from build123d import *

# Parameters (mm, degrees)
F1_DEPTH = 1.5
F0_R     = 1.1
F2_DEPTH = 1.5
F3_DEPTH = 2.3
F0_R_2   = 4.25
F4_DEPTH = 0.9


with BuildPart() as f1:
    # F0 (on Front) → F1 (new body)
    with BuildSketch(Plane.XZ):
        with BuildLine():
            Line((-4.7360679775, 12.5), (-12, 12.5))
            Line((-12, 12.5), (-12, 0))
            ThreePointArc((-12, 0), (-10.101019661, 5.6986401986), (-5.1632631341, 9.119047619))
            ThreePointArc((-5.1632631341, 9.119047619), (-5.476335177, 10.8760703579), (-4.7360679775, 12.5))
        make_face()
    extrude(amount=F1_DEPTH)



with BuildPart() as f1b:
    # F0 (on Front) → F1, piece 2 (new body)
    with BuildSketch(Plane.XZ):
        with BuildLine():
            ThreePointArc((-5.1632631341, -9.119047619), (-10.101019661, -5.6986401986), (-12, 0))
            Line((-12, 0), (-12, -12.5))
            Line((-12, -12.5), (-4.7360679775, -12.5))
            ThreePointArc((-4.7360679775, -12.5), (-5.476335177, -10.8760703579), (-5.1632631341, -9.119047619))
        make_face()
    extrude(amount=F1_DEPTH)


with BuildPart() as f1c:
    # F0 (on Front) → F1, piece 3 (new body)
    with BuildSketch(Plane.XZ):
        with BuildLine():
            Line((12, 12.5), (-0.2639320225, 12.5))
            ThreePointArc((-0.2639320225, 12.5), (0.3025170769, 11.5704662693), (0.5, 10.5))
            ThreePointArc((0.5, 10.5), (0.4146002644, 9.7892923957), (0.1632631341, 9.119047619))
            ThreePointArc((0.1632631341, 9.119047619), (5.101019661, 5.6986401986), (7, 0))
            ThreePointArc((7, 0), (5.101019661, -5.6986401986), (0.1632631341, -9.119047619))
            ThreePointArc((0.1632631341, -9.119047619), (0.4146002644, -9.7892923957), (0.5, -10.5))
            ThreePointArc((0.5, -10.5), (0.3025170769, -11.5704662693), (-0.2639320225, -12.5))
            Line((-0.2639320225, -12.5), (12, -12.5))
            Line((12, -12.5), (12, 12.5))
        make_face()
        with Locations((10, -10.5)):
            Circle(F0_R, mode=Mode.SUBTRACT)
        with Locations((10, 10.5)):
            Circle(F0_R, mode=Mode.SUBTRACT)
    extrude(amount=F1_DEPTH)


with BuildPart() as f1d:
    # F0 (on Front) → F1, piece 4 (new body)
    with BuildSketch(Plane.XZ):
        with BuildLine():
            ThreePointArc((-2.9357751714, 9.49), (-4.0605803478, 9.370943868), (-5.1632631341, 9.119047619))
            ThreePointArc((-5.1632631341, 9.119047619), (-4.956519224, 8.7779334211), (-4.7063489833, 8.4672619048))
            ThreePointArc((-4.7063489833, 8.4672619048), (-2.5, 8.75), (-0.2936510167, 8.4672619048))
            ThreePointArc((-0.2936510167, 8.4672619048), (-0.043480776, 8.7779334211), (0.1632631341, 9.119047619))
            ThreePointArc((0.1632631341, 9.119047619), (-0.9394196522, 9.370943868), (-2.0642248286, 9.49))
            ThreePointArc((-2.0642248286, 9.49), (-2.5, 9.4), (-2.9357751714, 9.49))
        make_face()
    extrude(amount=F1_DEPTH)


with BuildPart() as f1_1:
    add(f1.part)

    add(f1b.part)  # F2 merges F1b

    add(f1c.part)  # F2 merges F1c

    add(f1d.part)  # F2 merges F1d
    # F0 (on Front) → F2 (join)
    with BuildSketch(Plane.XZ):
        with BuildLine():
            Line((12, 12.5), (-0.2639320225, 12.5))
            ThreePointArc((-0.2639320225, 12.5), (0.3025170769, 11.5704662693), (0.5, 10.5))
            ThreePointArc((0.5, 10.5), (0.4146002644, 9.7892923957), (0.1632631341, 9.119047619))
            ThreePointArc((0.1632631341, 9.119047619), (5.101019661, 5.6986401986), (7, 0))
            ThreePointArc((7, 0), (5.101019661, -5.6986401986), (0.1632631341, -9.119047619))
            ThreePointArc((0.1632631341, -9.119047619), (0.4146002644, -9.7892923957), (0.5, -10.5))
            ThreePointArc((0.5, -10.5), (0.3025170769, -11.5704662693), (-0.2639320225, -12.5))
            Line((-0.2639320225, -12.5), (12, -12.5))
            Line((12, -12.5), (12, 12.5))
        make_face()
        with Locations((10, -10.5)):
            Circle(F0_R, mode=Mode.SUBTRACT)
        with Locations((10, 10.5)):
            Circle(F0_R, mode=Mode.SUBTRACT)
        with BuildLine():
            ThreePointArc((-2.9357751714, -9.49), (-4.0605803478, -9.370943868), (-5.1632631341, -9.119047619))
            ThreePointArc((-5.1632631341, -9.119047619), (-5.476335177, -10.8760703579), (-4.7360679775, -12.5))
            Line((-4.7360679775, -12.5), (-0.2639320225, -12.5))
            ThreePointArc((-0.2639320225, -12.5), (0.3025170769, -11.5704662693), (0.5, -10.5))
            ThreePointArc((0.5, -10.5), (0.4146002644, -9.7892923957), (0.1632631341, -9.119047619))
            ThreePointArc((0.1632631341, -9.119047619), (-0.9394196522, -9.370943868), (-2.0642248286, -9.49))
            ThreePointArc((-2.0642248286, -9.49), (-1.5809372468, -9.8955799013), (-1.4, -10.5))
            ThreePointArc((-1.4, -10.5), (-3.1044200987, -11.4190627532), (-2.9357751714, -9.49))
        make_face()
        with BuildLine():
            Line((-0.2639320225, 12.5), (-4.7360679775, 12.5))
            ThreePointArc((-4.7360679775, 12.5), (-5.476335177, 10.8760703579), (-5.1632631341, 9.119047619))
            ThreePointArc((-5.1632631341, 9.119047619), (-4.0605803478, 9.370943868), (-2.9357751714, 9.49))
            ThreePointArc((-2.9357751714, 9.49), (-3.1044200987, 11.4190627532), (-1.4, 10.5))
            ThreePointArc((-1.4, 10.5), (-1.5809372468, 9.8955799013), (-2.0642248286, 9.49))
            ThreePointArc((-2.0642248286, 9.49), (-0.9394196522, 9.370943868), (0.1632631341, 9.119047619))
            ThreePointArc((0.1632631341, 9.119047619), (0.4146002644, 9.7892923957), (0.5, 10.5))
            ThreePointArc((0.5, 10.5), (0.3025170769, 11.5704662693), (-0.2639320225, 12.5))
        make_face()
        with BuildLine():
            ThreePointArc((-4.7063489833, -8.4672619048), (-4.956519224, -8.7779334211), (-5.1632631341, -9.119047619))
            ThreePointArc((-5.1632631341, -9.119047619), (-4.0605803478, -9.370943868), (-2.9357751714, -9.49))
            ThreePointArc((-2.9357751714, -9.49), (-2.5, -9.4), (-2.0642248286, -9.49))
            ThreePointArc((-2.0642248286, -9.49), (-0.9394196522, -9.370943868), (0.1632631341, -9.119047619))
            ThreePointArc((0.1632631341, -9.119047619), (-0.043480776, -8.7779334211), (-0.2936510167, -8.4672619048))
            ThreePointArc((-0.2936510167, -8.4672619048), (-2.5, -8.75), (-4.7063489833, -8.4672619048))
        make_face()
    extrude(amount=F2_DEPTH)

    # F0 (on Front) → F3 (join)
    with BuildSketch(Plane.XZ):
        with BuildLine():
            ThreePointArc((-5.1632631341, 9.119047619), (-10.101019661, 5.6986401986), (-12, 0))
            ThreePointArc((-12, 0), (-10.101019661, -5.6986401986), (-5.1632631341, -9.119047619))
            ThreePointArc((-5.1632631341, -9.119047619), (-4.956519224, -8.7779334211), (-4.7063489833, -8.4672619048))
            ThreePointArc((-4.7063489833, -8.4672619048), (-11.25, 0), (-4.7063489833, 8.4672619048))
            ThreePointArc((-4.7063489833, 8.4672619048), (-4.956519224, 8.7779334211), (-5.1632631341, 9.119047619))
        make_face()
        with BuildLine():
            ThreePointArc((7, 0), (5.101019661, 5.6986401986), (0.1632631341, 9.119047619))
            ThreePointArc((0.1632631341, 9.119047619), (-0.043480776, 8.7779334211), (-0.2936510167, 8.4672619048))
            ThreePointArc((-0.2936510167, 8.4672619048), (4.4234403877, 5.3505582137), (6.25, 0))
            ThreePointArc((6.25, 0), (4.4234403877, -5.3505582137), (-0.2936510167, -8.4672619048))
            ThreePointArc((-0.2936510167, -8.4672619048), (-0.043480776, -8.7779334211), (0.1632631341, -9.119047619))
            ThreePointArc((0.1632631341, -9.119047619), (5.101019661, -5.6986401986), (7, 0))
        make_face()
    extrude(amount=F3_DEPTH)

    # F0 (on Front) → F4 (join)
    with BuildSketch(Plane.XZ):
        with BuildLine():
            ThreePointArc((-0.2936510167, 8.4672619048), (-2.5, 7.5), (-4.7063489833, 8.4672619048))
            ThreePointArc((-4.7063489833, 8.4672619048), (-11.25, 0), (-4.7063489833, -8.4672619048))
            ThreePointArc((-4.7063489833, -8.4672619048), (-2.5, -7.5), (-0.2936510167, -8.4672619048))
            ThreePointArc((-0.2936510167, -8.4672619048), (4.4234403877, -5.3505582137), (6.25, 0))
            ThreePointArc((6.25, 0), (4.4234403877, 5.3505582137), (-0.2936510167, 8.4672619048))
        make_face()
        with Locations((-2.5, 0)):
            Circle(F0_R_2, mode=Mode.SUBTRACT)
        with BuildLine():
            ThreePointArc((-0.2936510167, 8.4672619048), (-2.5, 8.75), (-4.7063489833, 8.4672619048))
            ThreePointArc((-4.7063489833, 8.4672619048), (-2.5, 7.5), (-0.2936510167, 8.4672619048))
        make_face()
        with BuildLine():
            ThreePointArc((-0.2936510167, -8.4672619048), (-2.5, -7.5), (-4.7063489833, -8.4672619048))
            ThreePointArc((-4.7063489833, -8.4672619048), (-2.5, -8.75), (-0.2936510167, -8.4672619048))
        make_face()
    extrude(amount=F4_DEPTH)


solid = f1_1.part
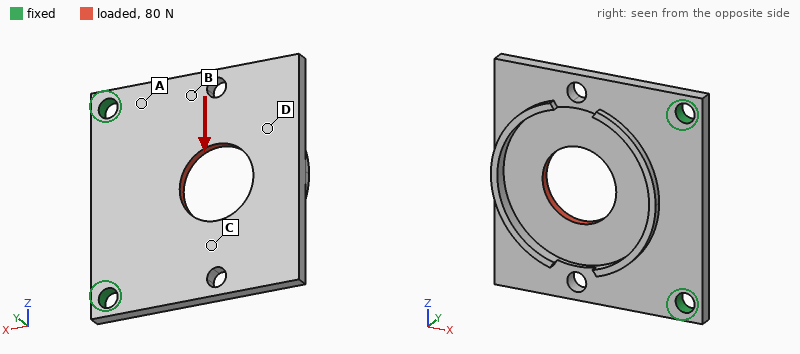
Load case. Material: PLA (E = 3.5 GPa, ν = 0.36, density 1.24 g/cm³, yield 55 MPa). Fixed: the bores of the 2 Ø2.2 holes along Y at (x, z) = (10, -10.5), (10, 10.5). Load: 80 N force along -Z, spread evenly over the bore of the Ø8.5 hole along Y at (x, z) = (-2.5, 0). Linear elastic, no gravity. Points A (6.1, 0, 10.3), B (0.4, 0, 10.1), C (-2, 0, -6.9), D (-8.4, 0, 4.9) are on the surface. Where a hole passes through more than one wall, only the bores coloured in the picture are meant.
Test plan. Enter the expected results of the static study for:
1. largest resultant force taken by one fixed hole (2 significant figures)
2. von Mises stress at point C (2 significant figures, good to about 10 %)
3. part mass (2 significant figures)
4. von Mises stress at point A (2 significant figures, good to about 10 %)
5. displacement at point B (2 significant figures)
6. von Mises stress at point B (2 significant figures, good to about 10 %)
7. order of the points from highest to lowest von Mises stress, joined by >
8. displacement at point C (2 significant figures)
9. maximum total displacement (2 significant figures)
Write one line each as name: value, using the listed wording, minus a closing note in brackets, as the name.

largest resultant force taken by one fixed hole: 60 N
von Mises stress at point C: 7.9 MPa
part mass: 0.88 g
von Mises stress at point A: 6.4 MPa
displacement at point B: 37 µm
von Mises stress at point B: 5.2 MPa
order of the points from highest to lowest von Mises stress, joined by >: C > A > B > D
displacement at point C: 50 µm
maximum total displacement: 86 µm
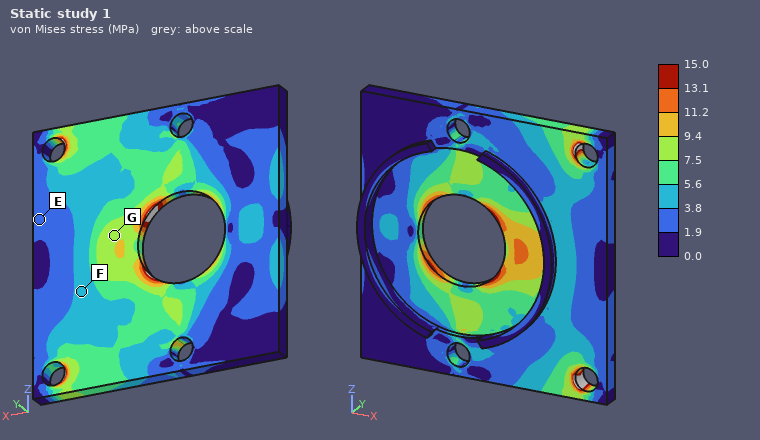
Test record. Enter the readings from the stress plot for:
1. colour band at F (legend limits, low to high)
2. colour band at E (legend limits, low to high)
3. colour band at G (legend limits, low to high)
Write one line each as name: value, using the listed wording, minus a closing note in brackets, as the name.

colour band at F: 3.8 to 5.6 MPa
colour band at E: 1.9 to 3.8 MPa
colour band at G: 7.5 to 9.4 MPa
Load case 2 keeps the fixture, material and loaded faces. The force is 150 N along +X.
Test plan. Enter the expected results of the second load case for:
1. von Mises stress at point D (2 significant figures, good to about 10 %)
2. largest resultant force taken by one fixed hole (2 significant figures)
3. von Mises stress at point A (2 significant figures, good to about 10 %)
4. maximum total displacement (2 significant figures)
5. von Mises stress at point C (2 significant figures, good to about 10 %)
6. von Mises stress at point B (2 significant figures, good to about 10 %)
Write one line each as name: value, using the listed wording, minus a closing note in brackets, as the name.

von Mises stress at point D: 5.6 MPa
largest resultant force taken by one fixed hole: 80 N
von Mises stress at point A: 14 MPa
maximum total displacement: 0.39 mm
von Mises stress at point C: 8.8 MPa
von Mises stress at point B: 6.6 MPa
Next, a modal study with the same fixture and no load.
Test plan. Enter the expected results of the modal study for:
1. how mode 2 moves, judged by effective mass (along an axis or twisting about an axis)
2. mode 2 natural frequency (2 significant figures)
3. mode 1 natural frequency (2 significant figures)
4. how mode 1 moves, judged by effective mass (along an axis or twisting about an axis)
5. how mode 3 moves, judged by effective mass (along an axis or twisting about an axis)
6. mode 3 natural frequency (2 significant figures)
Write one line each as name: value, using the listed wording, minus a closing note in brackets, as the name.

how mode 2 moves, judged by effective mass: twisting about X
mode 2 natural frequency: 1600 Hz
mode 1 natural frequency: 730 Hz
how mode 1 moves, judged by effective mass: along Y
how mode 3 moves, judged by effective mass: along Y
mode 3 natural frequency: 4000 Hz
